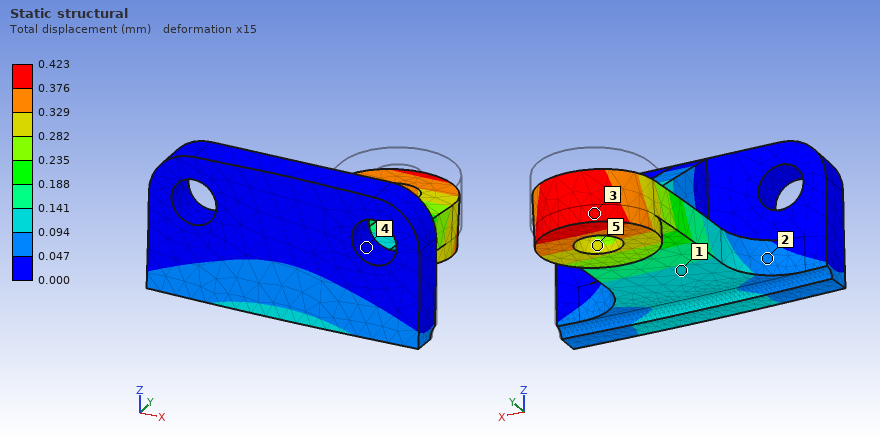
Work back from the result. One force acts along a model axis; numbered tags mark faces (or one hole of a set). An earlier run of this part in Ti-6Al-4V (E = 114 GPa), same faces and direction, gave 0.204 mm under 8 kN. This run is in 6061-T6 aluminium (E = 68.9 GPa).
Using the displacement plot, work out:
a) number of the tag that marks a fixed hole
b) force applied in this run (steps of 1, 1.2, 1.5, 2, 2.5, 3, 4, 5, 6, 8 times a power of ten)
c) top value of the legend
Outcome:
4
10 kN
0.423 mm
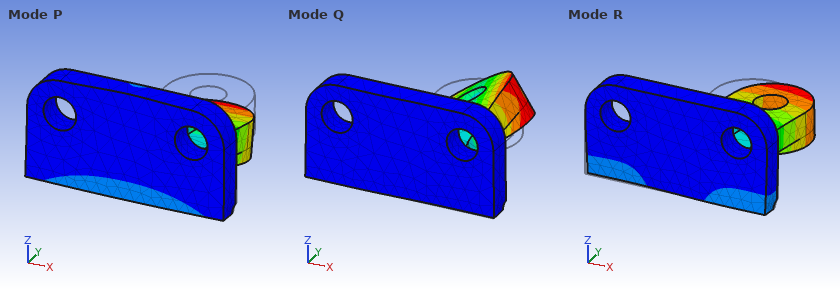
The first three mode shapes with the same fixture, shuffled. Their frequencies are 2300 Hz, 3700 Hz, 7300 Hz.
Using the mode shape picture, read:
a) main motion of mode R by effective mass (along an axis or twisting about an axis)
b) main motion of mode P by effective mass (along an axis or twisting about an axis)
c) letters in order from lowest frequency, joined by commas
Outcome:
along X
along Z
P, R, Q
